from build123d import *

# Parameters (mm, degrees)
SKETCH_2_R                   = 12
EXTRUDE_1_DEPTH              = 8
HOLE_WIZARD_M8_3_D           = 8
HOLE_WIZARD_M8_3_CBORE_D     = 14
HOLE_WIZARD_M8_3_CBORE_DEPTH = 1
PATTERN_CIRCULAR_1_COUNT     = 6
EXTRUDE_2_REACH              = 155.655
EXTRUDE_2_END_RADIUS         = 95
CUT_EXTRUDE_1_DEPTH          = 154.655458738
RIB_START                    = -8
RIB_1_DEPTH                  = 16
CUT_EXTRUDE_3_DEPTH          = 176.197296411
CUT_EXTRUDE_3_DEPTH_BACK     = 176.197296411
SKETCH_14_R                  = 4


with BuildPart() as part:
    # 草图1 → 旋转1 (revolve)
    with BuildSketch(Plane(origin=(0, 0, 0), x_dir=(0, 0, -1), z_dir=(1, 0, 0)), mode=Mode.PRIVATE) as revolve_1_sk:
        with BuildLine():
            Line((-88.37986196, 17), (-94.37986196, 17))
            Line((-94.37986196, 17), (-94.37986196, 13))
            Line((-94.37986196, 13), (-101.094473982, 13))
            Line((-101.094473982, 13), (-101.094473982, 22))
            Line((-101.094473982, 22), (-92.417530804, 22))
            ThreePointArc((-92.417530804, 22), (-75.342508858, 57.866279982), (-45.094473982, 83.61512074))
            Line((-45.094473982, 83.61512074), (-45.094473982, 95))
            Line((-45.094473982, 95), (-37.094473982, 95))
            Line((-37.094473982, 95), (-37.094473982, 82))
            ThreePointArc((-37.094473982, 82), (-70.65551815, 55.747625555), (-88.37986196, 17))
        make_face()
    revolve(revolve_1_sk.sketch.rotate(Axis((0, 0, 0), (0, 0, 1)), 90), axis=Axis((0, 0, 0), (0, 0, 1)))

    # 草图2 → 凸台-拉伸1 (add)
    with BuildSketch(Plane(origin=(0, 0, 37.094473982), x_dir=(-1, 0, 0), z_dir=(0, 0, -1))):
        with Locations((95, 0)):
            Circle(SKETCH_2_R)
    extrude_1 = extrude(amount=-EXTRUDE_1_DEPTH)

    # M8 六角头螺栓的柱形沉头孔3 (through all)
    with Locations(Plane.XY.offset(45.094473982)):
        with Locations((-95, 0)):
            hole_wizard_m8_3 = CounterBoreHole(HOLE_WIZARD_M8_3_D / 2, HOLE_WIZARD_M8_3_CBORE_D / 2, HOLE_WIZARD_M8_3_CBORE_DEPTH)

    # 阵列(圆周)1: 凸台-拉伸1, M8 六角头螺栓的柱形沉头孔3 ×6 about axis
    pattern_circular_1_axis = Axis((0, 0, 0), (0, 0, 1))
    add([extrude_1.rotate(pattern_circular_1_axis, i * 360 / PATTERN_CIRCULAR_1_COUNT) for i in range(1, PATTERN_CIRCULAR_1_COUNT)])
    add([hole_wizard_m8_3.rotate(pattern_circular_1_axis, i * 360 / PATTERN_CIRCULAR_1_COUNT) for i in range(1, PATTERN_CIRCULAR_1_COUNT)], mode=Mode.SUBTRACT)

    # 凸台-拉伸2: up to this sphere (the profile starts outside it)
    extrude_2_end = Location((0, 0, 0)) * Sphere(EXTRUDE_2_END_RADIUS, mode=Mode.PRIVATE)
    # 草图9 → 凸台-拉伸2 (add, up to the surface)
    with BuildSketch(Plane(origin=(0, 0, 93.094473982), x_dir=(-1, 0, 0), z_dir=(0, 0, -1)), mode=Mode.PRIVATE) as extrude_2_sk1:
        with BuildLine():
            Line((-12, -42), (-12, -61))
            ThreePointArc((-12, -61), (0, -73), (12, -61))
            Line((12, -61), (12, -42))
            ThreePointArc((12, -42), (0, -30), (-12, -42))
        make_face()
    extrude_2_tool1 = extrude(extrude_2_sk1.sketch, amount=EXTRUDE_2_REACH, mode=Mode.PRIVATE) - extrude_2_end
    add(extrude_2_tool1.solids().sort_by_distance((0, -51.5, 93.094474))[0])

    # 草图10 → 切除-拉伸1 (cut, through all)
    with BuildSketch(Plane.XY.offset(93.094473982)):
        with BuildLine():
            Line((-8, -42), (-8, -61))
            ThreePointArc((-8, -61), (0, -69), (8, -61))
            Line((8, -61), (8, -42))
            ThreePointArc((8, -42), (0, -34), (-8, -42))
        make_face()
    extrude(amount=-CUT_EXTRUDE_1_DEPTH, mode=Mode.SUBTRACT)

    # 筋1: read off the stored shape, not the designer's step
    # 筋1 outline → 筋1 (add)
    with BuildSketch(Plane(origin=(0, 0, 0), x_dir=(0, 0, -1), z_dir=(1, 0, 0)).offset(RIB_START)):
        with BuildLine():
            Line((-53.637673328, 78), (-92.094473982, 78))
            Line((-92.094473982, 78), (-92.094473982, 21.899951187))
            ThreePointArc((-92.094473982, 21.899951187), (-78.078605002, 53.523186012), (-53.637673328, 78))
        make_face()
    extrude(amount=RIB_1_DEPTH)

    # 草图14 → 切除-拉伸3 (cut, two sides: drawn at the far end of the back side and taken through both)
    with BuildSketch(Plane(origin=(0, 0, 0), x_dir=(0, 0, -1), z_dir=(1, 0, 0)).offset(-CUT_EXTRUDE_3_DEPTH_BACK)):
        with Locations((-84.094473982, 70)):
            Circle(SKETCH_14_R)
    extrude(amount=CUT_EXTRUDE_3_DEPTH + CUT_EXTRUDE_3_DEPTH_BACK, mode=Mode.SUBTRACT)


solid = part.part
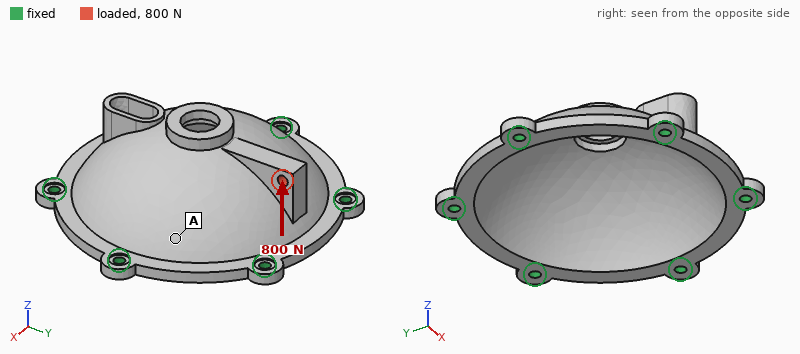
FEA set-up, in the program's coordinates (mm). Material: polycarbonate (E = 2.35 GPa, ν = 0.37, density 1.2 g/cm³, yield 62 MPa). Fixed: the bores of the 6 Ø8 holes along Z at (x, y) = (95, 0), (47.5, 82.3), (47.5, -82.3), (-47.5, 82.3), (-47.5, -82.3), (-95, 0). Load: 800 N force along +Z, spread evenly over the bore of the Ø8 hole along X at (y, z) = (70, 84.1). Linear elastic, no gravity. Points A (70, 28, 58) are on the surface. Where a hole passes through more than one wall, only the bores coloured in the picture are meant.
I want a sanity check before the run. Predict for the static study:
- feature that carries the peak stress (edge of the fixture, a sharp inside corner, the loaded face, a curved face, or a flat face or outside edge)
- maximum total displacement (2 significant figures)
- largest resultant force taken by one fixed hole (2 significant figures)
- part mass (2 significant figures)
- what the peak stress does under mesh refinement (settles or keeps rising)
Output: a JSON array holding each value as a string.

["edge of the fixture", "0.38 mm", "640 N", "280 g", "keeps rising"]
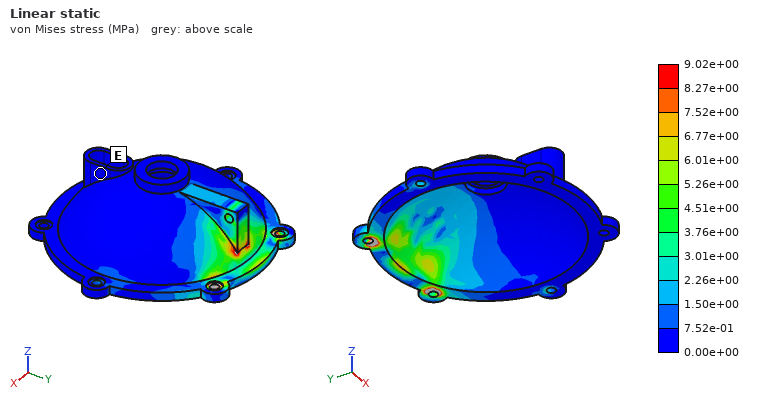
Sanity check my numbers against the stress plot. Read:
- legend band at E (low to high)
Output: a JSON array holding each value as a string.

["0.00e+00 to 7.52e-01 MPa"]
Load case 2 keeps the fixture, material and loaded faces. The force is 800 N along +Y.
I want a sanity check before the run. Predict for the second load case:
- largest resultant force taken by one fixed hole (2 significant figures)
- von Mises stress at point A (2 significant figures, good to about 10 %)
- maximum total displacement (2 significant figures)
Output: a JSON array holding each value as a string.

["220 N", "0.70 MPa", "0.22 mm"]
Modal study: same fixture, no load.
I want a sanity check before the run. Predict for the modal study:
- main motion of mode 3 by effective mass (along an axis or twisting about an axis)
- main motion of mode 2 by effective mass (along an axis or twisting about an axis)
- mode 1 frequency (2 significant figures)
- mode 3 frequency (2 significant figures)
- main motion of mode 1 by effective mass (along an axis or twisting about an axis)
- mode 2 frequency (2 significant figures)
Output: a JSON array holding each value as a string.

["along Z", "along Z", "1400 Hz", "1500 Hz", "along Z", "1400 Hz"]
